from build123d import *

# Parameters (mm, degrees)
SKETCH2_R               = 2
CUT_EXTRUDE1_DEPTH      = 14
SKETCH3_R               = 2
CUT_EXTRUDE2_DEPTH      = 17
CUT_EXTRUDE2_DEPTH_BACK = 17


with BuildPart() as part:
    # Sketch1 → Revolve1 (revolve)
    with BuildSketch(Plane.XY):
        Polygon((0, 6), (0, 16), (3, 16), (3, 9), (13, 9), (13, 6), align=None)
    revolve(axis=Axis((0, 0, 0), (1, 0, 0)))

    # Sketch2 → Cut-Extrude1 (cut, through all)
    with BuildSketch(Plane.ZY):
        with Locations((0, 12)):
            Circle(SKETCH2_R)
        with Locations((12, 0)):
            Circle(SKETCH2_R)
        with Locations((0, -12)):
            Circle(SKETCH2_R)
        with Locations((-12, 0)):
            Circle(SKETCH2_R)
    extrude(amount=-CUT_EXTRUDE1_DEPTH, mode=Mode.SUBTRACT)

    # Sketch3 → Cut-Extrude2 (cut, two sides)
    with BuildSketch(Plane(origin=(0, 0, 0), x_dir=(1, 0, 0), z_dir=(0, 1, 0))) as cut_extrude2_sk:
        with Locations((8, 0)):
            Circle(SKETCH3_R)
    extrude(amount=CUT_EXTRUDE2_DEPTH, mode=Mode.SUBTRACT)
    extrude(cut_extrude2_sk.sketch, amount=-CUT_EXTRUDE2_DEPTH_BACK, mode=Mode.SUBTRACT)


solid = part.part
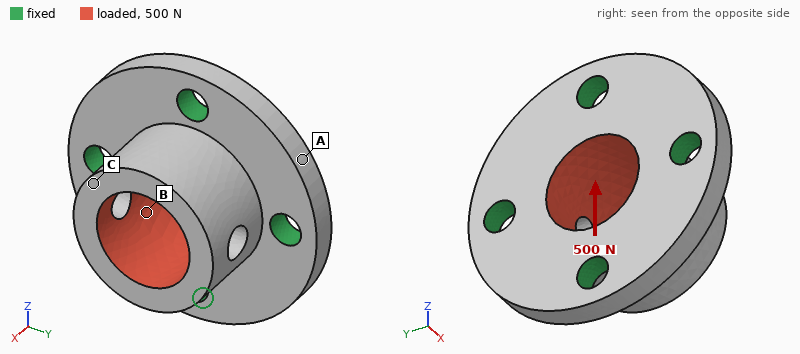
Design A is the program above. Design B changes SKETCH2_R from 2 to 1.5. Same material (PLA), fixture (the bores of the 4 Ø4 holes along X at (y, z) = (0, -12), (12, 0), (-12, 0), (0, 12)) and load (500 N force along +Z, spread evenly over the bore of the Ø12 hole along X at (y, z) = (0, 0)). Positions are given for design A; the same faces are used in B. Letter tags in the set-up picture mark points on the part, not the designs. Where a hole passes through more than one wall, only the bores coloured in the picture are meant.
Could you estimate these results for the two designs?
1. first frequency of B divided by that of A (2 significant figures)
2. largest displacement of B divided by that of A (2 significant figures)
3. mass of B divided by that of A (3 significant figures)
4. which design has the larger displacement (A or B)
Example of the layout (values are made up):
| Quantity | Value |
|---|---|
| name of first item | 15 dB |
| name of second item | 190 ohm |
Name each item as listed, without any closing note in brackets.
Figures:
| Quantity | Value |
|---|---|
| first frequency of B divided by that of A | 0.91 |
| largest displacement of B divided by that of A | 1.1 |
| mass of B divided by that of A | 1.02 |
| which design has the larger displacement | B |
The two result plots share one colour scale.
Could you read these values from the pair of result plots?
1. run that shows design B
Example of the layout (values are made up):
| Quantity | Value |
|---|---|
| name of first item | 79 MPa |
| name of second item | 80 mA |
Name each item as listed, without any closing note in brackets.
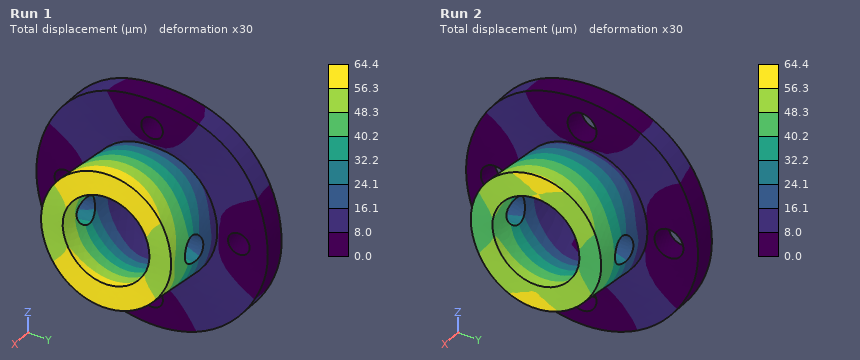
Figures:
| Quantity | Value |
|---|---|
| run that shows design B | Run 1 |
